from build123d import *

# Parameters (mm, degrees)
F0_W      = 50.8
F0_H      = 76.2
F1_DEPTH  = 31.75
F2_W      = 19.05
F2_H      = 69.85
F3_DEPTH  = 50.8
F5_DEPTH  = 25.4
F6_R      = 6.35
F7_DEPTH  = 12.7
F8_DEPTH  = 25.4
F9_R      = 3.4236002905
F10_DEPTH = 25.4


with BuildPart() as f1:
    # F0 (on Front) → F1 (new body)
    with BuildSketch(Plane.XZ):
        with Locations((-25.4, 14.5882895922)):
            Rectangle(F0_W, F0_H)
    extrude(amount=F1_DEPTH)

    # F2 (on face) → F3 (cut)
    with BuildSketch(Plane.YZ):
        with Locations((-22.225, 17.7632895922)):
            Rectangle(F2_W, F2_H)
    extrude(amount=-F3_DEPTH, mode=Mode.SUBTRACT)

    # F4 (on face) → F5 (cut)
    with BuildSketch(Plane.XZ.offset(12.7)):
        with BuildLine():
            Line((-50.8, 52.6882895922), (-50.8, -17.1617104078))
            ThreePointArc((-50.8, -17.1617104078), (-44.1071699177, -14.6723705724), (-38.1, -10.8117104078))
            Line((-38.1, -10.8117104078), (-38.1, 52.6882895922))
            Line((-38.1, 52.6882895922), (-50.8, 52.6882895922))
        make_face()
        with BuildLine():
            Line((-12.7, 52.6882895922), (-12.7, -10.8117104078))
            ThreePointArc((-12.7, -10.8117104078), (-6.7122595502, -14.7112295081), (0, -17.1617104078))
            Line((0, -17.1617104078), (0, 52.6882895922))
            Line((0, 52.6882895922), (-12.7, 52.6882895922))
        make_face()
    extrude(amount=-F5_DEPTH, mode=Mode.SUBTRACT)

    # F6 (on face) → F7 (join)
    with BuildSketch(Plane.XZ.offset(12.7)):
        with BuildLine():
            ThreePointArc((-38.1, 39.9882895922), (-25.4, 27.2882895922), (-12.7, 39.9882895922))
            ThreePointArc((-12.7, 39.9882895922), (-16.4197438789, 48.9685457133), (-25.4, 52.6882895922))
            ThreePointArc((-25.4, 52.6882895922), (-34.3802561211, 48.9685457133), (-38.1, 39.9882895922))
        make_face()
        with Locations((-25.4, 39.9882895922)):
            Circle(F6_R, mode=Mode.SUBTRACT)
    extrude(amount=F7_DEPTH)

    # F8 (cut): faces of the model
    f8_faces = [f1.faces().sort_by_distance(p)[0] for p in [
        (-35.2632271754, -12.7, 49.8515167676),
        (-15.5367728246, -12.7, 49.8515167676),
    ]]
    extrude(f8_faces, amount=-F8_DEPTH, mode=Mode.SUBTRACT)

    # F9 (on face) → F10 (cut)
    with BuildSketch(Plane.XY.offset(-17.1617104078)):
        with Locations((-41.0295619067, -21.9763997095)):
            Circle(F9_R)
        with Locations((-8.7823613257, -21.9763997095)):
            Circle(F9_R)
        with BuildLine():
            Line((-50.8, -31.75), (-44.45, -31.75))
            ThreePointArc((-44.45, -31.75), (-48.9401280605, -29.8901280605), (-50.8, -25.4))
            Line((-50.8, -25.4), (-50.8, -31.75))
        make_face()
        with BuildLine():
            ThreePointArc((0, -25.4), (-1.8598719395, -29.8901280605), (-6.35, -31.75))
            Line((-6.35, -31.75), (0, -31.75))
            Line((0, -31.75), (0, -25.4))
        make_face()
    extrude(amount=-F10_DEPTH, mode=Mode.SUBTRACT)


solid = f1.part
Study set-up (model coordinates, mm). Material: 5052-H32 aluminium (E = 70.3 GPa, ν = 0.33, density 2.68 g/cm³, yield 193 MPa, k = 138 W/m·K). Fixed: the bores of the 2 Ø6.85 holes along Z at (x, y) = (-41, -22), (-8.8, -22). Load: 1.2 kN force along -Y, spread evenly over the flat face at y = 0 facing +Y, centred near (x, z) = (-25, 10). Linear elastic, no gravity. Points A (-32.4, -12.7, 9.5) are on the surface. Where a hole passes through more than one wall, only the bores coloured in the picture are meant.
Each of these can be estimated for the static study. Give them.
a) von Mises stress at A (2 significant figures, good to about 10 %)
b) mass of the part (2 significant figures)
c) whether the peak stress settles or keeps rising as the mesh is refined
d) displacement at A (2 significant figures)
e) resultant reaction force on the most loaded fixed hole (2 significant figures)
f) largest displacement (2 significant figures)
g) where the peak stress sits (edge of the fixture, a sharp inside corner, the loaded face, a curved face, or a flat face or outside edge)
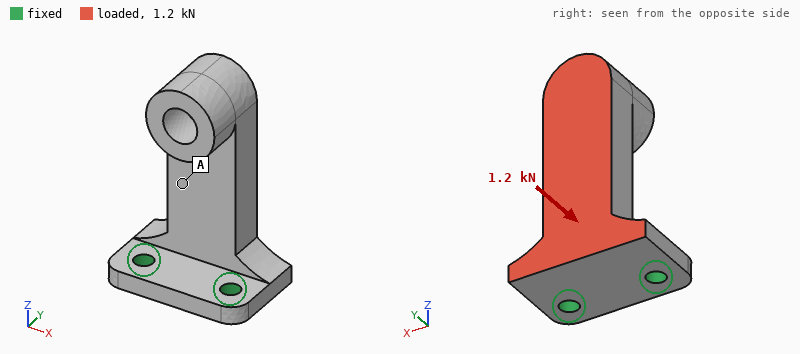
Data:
17 MPa
99 g
keeps rising
0.20 mm
660 N
0.54 mm
edge of the fixture
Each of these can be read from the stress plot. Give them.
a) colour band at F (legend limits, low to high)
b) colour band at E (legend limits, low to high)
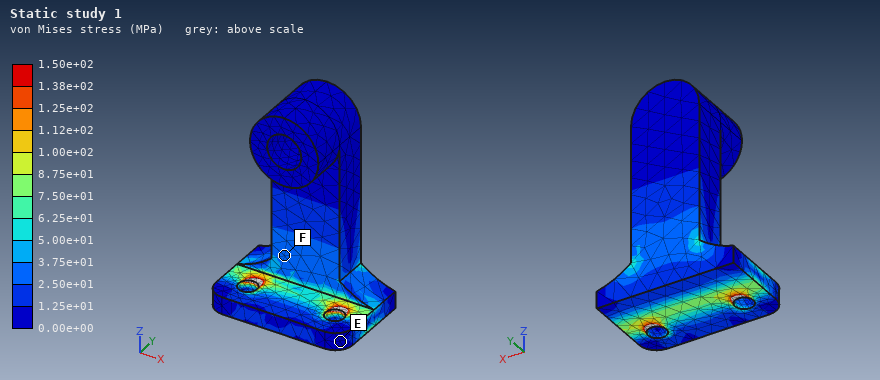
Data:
2.50e+01 to 3.75e+01 MPa
0.00e+00 to 1.25e+01 MPa
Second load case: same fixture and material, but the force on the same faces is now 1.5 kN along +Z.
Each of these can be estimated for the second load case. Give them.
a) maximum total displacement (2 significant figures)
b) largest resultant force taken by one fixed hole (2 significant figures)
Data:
0.31 mm
770 N
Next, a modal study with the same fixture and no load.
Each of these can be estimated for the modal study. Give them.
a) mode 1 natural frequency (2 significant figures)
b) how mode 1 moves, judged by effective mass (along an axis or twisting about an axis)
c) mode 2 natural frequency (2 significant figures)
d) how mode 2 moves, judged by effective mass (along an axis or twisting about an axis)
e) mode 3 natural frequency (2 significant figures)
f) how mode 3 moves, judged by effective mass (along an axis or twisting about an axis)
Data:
900 Hz
along Y
2100 Hz
along X
5100 Hz
along Z
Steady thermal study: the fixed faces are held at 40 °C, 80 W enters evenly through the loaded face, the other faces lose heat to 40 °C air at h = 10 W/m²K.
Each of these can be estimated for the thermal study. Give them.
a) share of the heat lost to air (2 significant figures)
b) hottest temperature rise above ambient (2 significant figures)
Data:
4.4 %
73 K
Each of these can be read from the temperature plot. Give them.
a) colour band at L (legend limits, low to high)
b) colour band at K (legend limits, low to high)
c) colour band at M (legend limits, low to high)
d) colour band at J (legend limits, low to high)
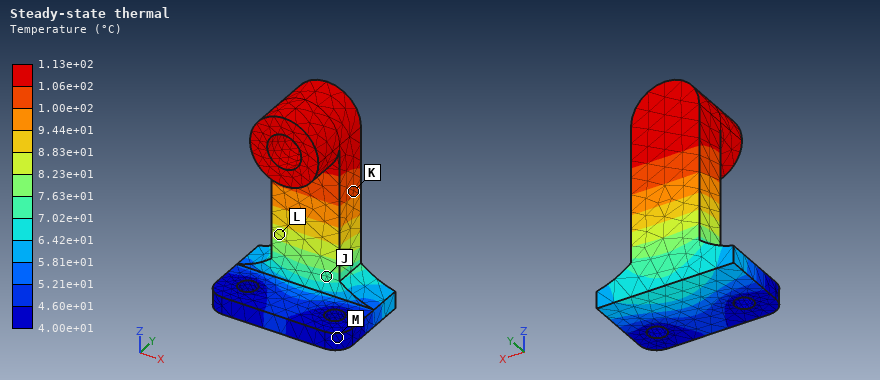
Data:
8.23e+01 to 8.83e+01 °C
1.00e+02 to 1.06e+02 °C
4.00e+01 to 4.60e+01 °C
7.02e+01 to 7.63e+01 °C
